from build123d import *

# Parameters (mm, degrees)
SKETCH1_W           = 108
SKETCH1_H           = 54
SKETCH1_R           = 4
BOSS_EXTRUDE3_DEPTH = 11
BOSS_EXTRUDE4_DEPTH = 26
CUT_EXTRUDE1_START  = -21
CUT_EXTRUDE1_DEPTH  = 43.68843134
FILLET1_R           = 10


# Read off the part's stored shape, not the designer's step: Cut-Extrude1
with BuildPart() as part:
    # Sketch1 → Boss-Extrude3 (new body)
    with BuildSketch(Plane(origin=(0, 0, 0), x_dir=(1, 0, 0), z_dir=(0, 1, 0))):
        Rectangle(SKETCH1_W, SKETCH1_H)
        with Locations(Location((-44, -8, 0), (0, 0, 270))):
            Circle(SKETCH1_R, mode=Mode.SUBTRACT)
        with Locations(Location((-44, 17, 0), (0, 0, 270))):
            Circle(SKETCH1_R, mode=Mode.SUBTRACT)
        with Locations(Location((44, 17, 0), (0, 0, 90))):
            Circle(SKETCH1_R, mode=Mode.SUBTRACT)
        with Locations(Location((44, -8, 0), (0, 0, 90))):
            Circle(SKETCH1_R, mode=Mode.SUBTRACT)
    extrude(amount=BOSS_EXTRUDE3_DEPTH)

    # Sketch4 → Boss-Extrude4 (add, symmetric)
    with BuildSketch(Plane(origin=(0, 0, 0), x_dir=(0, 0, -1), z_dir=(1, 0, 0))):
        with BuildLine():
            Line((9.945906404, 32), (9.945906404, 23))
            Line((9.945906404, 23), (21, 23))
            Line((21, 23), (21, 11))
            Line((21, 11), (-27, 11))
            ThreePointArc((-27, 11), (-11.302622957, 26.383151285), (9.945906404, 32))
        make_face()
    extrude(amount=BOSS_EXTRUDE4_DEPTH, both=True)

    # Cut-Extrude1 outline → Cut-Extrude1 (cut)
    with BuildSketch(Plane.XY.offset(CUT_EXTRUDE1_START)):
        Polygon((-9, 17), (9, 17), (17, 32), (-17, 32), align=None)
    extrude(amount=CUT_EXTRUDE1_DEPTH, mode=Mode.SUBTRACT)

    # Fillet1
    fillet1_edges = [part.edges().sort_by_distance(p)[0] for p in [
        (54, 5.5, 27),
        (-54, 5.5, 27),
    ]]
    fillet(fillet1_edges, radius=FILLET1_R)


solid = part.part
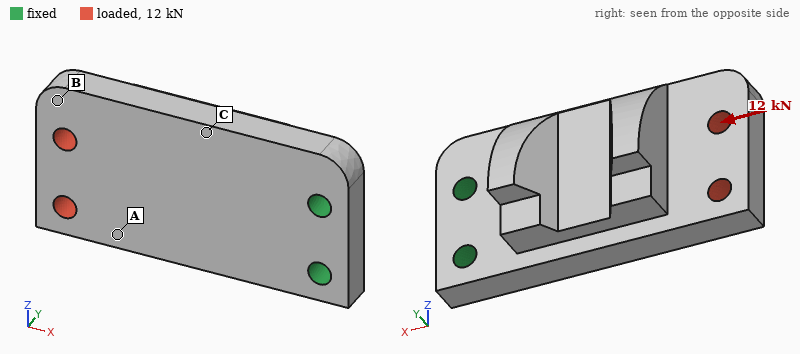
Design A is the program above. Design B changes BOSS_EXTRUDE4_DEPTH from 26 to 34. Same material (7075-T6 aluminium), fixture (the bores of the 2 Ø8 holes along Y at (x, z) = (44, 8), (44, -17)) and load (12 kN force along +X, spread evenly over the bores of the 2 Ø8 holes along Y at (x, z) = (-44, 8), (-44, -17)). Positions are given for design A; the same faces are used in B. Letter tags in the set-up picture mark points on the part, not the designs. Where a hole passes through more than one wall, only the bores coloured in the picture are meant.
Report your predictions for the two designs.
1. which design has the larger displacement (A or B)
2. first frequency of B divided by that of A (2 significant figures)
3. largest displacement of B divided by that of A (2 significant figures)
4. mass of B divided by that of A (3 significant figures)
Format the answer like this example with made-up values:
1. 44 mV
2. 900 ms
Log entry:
1. B
2. 1.0
3. 1.2
4. 1.13
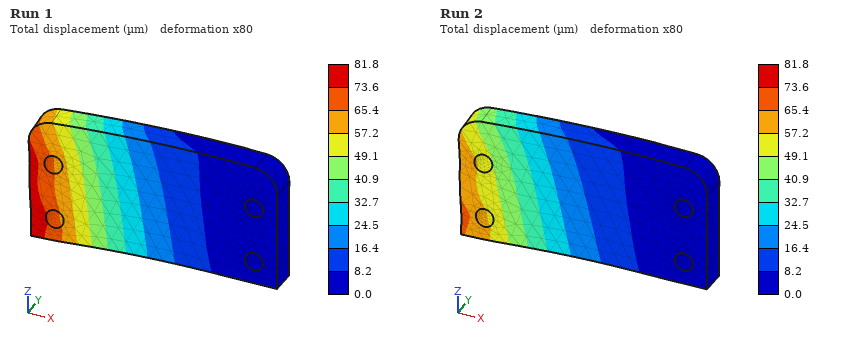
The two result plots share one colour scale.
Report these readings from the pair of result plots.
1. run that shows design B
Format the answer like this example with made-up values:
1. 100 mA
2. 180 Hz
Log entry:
1. Run 1
